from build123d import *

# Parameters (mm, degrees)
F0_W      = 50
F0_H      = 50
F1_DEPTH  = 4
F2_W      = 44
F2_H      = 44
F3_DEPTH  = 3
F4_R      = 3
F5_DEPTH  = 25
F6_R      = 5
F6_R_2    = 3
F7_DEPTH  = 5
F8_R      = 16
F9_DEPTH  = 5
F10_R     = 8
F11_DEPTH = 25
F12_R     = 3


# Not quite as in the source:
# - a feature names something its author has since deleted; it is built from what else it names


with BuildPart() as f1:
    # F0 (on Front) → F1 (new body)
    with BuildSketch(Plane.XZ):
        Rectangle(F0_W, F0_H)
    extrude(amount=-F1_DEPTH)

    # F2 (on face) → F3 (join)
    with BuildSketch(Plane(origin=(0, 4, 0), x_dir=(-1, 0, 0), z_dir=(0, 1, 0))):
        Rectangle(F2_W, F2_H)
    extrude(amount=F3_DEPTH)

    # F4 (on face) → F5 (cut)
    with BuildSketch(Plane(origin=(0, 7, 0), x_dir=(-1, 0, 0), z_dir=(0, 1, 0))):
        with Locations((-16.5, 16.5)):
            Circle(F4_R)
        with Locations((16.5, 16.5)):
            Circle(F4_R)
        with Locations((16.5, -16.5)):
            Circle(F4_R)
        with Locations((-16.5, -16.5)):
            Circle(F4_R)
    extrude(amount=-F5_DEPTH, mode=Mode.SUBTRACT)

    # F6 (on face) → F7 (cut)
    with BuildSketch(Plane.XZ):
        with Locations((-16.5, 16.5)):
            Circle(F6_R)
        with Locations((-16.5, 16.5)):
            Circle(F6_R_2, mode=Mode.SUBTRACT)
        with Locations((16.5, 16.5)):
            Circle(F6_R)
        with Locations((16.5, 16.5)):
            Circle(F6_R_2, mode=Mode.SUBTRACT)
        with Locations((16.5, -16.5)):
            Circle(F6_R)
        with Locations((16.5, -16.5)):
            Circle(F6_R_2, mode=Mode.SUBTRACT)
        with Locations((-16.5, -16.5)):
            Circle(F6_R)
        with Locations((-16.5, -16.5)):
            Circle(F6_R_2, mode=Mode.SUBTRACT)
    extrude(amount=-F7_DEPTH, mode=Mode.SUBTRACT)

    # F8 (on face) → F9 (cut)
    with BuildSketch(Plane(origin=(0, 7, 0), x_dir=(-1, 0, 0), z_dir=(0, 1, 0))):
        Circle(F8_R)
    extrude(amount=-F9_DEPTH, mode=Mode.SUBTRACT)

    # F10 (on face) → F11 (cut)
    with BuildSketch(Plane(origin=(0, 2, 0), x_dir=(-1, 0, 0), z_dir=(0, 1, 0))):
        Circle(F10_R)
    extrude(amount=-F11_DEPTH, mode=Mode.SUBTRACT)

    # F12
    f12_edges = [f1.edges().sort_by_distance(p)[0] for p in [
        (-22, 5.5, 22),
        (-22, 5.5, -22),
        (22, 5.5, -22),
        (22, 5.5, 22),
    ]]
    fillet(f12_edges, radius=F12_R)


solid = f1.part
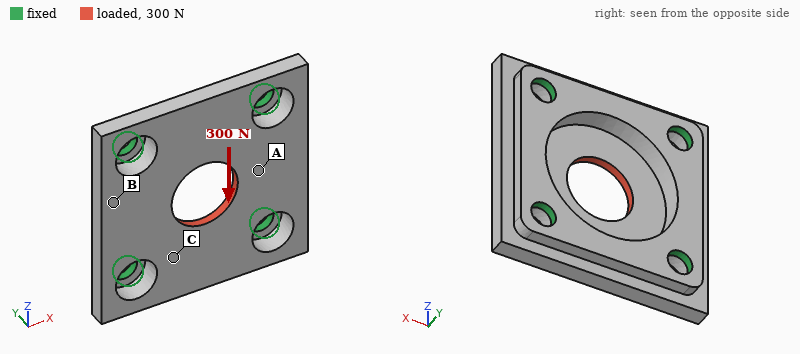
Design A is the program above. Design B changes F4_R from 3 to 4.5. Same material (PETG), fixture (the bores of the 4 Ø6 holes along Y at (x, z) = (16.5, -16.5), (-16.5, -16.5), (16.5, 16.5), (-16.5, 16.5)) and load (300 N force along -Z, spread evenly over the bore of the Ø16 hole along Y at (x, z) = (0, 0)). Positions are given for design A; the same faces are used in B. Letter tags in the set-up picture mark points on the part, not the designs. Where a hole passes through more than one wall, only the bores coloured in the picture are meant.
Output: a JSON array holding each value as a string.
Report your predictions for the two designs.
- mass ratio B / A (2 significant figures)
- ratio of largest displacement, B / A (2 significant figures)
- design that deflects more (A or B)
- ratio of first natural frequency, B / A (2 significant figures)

["0.97", "0.80", "A", "1.2"]
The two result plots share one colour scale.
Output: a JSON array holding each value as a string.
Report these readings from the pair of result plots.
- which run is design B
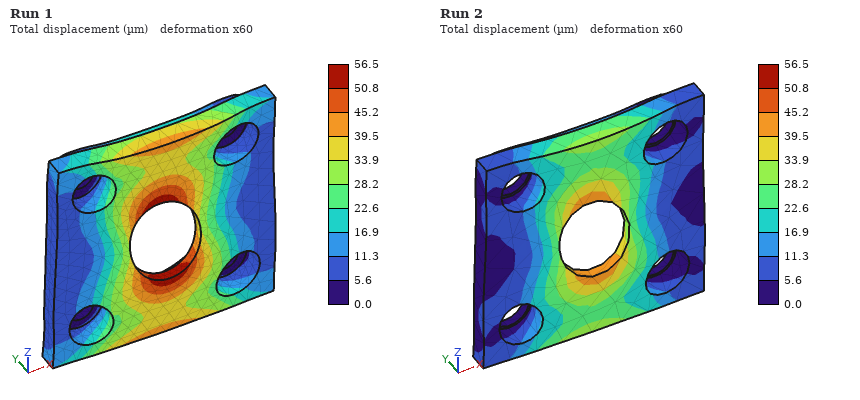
["Run 2"]
